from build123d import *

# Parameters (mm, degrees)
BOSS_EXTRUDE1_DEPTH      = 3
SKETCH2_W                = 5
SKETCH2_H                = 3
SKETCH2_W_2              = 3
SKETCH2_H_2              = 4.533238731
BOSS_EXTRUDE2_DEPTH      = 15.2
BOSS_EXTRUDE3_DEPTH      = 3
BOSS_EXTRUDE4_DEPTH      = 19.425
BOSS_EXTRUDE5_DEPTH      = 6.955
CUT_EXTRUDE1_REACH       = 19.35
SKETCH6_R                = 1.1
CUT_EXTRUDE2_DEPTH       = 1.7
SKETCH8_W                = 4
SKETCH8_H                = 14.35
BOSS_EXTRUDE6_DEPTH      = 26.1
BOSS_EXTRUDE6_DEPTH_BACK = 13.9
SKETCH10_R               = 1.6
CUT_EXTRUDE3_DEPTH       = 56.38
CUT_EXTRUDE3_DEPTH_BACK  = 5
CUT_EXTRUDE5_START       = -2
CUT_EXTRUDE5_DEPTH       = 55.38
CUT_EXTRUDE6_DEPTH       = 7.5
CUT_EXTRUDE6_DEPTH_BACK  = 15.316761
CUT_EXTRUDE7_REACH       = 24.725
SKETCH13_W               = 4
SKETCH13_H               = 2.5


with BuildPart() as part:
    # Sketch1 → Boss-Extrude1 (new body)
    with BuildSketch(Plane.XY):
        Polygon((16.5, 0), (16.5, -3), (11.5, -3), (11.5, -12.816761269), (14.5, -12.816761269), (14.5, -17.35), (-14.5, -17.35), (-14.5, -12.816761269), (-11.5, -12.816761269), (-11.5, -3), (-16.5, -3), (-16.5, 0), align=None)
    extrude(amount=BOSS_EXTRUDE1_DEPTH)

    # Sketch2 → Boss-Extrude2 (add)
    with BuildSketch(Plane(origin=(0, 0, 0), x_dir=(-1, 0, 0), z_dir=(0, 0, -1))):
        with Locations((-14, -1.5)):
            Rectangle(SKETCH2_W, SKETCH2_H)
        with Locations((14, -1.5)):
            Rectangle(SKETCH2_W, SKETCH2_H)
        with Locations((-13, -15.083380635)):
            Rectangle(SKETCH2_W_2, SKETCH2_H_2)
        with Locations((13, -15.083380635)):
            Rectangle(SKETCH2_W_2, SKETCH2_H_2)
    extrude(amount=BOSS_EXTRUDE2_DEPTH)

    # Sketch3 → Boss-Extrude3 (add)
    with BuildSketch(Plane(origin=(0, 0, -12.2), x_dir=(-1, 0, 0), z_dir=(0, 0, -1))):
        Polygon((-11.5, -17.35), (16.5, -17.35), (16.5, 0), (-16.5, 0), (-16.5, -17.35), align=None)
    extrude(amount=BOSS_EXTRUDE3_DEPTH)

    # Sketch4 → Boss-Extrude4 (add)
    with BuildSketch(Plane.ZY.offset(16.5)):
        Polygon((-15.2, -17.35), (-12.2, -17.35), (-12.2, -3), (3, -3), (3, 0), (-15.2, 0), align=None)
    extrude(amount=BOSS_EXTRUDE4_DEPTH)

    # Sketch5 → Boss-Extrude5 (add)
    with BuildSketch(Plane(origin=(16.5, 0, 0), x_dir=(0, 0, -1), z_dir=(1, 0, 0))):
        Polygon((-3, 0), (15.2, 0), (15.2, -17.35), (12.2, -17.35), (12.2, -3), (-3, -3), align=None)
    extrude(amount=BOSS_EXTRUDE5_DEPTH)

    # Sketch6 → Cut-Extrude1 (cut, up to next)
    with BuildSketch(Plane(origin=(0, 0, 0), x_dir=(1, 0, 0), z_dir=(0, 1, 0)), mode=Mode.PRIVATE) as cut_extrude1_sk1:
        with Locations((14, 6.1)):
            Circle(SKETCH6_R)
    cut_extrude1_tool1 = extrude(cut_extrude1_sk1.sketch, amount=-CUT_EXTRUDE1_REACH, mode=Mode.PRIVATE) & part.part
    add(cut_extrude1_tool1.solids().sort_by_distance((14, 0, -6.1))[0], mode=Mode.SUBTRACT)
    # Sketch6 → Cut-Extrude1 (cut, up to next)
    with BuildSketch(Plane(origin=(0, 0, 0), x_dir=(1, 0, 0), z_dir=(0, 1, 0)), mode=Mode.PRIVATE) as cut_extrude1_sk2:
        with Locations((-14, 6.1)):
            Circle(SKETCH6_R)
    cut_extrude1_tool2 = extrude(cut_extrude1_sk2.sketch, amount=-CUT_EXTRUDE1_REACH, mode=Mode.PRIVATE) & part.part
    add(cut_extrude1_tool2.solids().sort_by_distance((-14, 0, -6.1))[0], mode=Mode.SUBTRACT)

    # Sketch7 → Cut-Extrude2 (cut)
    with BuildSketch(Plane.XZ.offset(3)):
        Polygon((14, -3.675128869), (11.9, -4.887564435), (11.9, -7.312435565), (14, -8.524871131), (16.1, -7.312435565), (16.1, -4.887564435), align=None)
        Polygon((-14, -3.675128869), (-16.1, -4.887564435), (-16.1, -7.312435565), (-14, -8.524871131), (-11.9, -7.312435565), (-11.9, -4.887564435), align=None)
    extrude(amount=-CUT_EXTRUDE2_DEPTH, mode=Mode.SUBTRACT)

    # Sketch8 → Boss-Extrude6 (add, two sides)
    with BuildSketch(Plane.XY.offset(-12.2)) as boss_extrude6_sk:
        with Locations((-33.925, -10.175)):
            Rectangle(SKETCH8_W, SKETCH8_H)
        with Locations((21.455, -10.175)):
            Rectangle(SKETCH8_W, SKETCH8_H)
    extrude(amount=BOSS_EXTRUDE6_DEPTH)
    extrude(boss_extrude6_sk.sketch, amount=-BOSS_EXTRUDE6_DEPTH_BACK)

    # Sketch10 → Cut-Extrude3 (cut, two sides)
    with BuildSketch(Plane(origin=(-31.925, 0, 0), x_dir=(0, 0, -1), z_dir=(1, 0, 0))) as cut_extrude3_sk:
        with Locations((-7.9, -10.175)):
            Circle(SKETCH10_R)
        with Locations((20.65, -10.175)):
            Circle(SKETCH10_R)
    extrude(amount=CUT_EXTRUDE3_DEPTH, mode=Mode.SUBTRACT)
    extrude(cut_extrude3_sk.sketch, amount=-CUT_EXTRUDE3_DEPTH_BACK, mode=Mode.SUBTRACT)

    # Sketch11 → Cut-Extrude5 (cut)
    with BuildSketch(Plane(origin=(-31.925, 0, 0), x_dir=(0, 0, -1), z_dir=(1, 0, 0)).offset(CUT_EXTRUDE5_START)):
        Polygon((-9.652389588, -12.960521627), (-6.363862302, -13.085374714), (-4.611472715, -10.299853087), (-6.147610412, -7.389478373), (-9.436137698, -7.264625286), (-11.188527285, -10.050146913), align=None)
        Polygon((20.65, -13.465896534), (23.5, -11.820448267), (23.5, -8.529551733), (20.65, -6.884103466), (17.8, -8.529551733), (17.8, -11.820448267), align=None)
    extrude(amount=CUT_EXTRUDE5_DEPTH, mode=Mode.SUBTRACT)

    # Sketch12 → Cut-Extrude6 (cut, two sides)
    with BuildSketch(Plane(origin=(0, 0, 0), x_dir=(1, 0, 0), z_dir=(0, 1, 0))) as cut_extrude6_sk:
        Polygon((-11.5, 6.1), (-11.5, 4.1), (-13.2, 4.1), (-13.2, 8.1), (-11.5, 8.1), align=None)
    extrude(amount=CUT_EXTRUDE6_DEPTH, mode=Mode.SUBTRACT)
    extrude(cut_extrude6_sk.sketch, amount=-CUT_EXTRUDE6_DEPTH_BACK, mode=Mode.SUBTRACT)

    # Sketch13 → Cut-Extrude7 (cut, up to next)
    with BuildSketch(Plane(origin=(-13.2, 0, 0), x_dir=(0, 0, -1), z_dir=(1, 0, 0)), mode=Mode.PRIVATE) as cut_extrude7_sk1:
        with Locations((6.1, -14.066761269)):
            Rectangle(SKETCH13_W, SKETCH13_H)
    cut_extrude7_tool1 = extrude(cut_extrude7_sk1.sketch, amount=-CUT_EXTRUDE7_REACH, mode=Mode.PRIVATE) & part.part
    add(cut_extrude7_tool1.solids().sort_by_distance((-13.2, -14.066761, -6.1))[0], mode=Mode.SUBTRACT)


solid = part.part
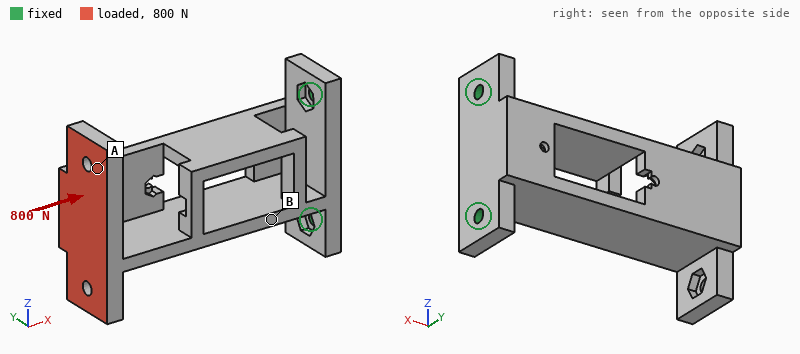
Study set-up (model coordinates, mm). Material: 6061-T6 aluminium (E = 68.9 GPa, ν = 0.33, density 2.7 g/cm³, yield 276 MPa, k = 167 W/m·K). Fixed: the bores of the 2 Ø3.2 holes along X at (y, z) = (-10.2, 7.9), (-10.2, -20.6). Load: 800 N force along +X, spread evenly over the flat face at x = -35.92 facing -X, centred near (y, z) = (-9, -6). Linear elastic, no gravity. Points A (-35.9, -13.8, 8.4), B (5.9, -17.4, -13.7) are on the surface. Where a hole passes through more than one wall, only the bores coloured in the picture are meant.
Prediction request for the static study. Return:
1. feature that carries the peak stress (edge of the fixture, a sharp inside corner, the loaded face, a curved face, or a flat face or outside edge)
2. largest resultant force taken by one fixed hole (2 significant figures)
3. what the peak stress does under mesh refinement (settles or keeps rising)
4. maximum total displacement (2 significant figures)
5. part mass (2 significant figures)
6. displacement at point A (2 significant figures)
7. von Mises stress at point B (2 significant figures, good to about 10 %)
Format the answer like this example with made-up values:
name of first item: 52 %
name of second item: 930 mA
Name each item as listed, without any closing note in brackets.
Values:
feature that carries the peak stress: edge of the fixture
largest resultant force taken by one fixed hole: 520 N
what the peak stress does under mesh refinement: keeps rising
maximum total displacement: 0.28 mm
part mass: 28 g
displacement at point A: 0.23 mm
von Mises stress at point B: 29 MPa
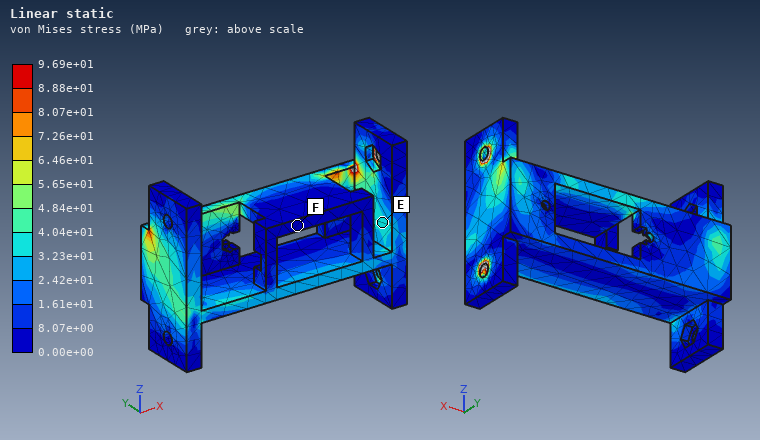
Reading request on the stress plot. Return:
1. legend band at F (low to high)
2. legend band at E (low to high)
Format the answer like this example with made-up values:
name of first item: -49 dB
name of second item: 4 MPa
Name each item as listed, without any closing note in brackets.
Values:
legend band at F: 0.00e+00 to 8.07e+00 MPa
legend band at E: 3.23e+01 to 4.04e+01 MPa
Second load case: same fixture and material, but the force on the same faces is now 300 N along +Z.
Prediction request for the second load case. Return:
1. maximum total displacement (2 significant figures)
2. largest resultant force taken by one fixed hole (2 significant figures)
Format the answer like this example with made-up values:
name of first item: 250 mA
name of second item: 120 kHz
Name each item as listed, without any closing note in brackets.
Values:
maximum total displacement: 0.69 mm
largest resultant force taken by one fixed hole: 740 N
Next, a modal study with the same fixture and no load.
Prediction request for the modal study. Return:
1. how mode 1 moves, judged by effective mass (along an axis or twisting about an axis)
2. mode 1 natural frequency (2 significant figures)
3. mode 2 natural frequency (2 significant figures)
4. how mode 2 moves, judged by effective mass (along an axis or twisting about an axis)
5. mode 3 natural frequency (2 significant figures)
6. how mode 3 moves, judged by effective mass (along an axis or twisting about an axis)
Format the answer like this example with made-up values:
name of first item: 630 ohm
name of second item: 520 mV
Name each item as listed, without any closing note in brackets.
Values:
how mode 1 moves, judged by effective mass: along Y
mode 1 natural frequency: 740 Hz
mode 2 natural frequency: 1100 Hz
how mode 2 moves, judged by effective mass: along Z
mode 3 natural frequency: 2600 Hz
how mode 3 moves, judged by effective mass: twisting about X
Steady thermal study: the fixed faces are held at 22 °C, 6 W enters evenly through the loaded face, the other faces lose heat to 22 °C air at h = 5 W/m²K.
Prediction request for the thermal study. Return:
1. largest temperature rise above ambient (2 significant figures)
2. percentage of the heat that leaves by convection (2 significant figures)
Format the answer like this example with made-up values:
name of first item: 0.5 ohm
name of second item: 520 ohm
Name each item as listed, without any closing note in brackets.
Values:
largest temperature rise above ambient: 28 K
percentage of the heat that leaves by convection: 7.9 %
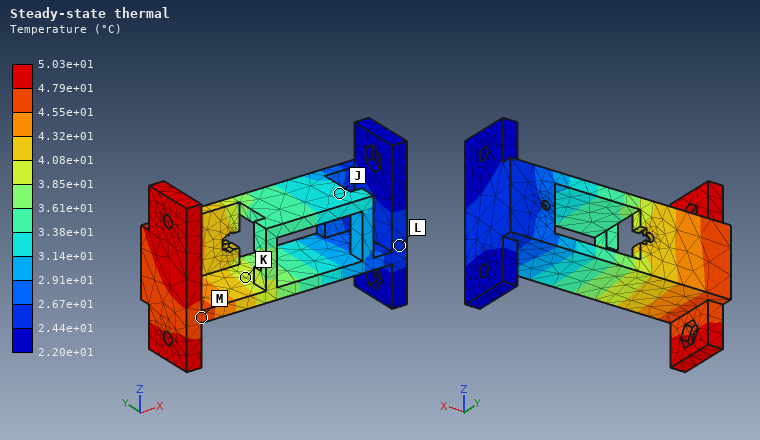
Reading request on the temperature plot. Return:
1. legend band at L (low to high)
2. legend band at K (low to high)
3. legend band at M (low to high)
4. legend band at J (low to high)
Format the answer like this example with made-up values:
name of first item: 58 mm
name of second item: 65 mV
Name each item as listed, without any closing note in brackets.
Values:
legend band at L: 2.44e+01 to 2.67e+01 °C
legend band at K: 3.85e+01 to 4.08e+01 °C
legend band at M: 4.55e+01 to 4.79e+01 °C
legend band at J: 3.14e+01 to 3.38e+01 °C
